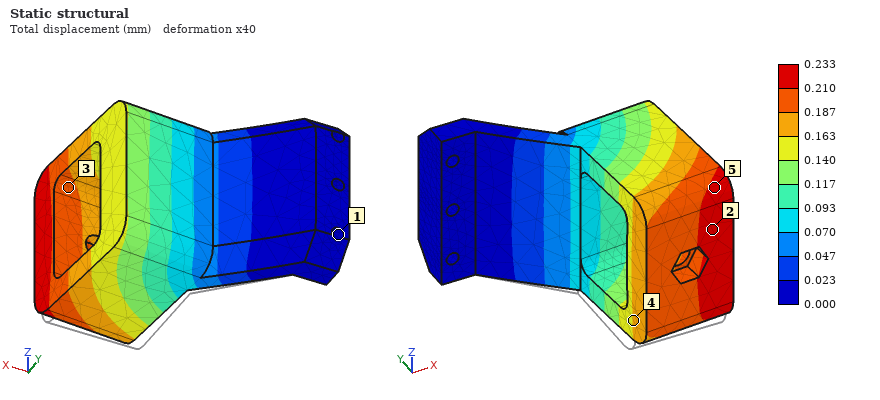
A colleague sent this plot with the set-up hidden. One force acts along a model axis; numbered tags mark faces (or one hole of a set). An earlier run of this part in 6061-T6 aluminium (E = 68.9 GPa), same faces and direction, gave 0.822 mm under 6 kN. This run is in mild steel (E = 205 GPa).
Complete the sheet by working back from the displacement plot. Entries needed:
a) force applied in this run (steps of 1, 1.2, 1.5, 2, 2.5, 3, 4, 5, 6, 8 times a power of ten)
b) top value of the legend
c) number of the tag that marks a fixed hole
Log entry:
5 kN
0.233 mm
1
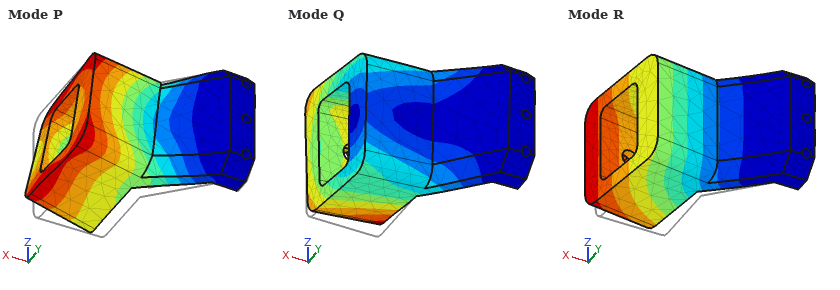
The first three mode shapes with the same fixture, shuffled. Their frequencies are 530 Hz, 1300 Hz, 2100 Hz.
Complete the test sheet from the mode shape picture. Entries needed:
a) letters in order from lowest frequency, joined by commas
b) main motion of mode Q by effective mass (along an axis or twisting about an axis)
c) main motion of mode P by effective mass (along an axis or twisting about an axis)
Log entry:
R, Q, P
along Z
along Z
